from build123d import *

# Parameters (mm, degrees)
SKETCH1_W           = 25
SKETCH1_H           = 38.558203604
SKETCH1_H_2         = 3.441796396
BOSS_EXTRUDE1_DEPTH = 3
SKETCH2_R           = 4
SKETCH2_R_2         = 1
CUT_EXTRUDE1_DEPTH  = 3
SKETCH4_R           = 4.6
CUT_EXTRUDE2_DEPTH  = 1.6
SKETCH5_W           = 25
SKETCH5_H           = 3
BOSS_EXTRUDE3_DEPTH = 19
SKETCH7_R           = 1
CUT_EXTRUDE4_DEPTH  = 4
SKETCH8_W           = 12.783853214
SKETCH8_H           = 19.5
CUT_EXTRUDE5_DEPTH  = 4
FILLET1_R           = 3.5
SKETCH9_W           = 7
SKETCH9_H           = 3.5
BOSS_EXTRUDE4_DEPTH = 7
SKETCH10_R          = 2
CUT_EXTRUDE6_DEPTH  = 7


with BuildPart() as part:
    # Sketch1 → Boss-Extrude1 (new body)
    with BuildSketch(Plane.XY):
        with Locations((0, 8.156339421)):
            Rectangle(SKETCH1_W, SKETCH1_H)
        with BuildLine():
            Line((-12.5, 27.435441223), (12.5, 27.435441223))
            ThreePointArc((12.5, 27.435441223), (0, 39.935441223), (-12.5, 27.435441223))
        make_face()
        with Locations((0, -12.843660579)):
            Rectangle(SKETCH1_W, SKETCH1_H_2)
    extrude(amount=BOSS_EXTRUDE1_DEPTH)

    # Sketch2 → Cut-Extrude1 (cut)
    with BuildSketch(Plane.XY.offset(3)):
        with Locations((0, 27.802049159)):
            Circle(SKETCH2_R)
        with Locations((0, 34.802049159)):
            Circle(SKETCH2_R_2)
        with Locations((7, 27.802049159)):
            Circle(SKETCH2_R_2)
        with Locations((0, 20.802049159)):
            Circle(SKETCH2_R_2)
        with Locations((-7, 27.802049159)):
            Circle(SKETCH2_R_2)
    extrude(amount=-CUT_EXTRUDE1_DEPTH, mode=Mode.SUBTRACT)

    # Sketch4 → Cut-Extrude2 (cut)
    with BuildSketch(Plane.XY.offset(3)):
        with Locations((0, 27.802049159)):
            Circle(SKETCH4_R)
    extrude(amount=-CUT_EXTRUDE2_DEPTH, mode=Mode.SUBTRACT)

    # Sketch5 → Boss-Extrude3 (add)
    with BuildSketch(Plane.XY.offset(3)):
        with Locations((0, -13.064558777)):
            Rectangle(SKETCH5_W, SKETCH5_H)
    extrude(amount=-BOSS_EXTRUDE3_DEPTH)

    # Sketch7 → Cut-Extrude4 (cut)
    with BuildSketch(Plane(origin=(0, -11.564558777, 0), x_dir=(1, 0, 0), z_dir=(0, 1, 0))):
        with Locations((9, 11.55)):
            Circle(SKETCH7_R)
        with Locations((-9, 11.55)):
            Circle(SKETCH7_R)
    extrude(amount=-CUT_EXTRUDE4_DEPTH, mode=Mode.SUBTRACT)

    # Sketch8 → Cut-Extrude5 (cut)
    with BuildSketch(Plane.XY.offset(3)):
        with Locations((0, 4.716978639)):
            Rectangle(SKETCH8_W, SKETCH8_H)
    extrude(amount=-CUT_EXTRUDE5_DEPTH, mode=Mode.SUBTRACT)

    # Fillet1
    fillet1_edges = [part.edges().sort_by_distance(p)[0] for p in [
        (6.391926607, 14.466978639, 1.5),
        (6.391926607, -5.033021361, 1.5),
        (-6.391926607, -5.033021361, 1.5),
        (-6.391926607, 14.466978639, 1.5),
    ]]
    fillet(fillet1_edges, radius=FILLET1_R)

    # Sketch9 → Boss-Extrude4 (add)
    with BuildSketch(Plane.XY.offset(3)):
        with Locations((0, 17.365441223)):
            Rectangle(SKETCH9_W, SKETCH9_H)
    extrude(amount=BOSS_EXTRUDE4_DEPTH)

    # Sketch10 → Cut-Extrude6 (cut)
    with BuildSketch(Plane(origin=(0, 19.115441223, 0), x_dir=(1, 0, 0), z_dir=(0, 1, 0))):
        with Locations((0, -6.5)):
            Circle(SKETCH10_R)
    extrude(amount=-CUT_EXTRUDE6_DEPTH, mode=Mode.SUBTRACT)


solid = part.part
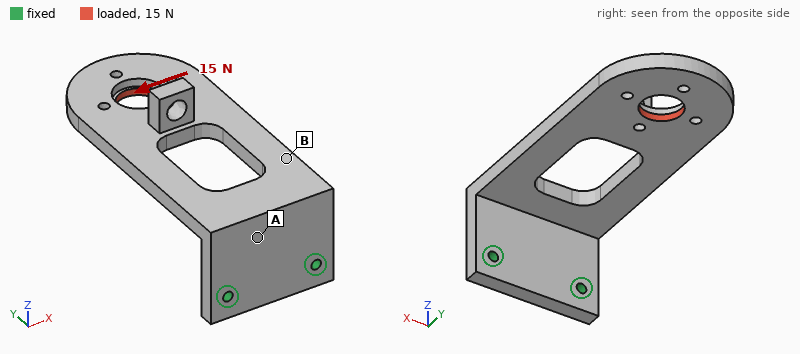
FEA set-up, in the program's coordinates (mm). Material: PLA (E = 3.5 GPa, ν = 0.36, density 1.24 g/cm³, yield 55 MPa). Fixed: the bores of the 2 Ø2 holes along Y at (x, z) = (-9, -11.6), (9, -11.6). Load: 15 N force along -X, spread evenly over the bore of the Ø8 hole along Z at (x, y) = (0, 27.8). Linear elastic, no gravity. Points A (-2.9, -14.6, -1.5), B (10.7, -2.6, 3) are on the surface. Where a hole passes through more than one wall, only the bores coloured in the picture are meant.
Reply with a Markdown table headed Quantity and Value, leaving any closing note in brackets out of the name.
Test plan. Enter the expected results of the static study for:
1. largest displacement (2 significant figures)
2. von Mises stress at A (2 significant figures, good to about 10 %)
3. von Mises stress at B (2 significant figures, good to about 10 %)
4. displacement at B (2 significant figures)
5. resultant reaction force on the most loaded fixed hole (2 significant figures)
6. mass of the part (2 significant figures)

| Quantity | Value |
|---|---|
| largest displacement | 0.74 mm |
| von Mises stress at A | 6.8 MPa |
| von Mises stress at B | 1.3 MPa |
| displacement at B | 0.20 mm |
| resultant reaction force on the most loaded fixed hole | 35 N |
| mass of the part | 5.3 g |
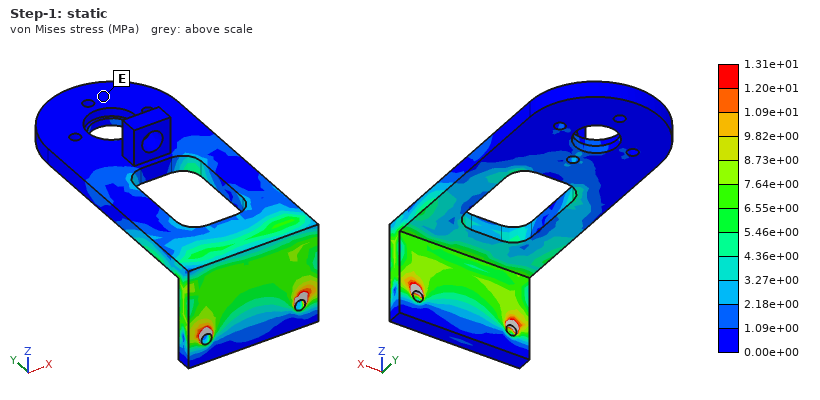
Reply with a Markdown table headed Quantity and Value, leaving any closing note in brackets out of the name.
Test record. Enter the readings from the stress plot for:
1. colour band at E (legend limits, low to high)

| Quantity | Value |
|---|---|
| colour band at E | 0.00e+00 to 1.09e+00 MPa |
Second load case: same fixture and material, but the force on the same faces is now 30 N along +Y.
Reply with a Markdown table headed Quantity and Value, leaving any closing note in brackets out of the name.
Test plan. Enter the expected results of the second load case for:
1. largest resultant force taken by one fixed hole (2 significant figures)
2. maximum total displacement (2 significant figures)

| Quantity | Value |
|---|---|
| largest resultant force taken by one fixed hole | 15 N |
| maximum total displacement | 0.46 mm |
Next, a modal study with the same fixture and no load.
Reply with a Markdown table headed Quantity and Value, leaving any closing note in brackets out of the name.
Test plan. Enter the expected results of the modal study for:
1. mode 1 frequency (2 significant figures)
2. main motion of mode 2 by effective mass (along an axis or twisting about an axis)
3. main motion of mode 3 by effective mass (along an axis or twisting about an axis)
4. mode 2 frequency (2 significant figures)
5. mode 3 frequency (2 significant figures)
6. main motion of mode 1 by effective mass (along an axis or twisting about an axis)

| Quantity | Value |
|---|---|
| mode 1 frequency | 210 Hz |
| main motion of mode 2 by effective mass | along X |
| main motion of mode 3 by effective mass | twisting about Y |
| mode 2 frequency | 560 Hz |
| mode 3 frequency | 1100 Hz |
| main motion of mode 1 by effective mass | along Z |
